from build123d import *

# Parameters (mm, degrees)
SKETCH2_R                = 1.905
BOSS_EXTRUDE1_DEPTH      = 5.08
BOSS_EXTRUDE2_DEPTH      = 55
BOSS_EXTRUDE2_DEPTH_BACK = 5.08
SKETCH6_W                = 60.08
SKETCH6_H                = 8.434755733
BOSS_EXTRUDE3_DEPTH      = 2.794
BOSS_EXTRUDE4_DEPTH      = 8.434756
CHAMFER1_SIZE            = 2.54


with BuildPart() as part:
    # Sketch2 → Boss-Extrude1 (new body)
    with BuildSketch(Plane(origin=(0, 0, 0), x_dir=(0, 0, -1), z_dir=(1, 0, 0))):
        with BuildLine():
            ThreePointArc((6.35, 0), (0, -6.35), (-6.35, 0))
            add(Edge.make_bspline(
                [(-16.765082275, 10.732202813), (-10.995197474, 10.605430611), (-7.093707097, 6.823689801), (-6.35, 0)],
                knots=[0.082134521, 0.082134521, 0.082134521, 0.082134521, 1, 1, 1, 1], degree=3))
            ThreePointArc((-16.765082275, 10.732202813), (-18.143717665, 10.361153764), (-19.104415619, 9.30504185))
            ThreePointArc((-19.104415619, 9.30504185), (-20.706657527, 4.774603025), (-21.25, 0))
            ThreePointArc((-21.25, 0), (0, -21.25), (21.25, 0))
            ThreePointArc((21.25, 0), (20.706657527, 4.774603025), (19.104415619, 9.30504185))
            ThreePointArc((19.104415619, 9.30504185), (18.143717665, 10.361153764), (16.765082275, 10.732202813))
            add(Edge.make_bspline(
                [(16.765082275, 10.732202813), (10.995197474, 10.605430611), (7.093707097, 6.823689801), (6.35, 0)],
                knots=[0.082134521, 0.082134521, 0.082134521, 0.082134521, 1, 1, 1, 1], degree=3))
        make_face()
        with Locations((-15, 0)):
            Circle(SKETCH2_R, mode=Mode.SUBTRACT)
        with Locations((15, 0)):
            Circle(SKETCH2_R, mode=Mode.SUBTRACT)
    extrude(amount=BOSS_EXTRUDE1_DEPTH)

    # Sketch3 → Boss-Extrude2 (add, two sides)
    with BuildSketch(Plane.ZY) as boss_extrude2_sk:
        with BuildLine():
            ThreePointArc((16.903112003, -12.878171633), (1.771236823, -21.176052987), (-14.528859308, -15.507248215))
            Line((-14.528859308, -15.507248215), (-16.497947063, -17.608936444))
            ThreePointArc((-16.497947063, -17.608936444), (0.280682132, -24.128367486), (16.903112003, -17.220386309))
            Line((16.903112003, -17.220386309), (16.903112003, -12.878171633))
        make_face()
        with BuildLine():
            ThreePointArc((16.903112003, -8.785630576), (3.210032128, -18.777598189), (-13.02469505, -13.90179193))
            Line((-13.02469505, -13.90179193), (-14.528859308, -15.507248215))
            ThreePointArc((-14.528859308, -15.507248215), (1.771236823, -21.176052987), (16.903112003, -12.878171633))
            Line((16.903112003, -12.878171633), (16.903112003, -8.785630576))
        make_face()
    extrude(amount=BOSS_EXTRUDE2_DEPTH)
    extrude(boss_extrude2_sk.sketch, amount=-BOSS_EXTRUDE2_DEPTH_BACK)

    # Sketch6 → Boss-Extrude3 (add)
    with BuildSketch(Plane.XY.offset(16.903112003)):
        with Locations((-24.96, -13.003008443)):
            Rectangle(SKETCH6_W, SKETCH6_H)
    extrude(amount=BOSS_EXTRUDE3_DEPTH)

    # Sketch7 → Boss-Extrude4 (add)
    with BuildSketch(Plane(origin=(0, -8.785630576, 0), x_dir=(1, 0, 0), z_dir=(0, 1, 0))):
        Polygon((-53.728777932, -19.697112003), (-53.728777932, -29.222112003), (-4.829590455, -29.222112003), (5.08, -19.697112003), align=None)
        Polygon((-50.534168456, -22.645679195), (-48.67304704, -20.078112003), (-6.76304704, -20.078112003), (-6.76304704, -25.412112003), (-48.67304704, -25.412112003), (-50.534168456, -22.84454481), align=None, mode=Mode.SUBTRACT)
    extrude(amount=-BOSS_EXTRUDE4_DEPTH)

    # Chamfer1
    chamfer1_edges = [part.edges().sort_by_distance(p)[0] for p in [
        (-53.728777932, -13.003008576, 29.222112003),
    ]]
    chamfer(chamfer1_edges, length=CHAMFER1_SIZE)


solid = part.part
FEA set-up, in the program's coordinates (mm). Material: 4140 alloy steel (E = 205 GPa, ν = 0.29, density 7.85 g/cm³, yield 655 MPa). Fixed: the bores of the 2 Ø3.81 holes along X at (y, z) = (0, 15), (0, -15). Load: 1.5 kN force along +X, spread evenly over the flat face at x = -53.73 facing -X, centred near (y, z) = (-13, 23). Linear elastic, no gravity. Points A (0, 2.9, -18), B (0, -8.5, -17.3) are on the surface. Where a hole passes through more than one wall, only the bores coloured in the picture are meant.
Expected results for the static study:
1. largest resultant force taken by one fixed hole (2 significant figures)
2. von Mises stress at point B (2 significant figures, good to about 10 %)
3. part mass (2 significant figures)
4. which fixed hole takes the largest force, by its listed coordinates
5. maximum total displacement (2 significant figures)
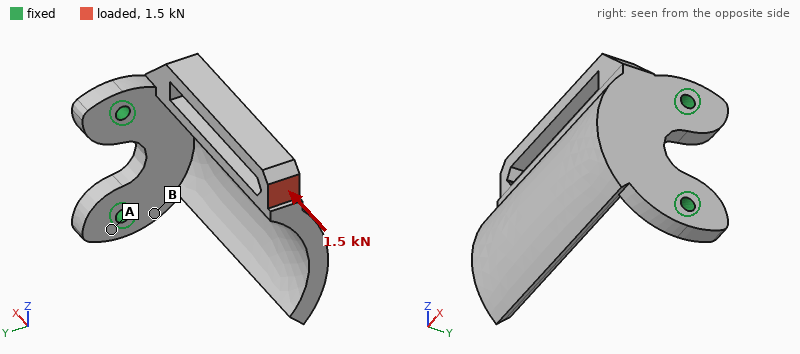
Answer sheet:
1.8 kN
48 MPa
150 g
(0, 15)
0.17 mm
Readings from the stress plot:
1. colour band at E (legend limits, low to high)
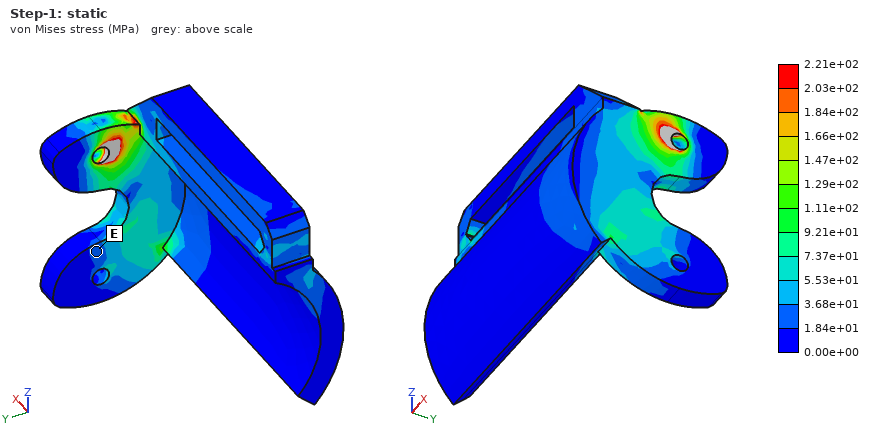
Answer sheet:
1.84e+01 to 3.68e+01 MPa
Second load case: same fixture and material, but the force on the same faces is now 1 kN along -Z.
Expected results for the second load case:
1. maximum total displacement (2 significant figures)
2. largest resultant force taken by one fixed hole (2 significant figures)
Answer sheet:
0.28 mm
1.8 kN
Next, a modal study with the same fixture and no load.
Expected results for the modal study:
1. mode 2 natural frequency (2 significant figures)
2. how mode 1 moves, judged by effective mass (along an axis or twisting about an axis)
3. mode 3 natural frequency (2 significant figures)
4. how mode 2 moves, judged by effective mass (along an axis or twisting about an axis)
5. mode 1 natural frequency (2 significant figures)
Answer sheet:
1900 Hz
along Y
3800 Hz
along Z
840 Hz
